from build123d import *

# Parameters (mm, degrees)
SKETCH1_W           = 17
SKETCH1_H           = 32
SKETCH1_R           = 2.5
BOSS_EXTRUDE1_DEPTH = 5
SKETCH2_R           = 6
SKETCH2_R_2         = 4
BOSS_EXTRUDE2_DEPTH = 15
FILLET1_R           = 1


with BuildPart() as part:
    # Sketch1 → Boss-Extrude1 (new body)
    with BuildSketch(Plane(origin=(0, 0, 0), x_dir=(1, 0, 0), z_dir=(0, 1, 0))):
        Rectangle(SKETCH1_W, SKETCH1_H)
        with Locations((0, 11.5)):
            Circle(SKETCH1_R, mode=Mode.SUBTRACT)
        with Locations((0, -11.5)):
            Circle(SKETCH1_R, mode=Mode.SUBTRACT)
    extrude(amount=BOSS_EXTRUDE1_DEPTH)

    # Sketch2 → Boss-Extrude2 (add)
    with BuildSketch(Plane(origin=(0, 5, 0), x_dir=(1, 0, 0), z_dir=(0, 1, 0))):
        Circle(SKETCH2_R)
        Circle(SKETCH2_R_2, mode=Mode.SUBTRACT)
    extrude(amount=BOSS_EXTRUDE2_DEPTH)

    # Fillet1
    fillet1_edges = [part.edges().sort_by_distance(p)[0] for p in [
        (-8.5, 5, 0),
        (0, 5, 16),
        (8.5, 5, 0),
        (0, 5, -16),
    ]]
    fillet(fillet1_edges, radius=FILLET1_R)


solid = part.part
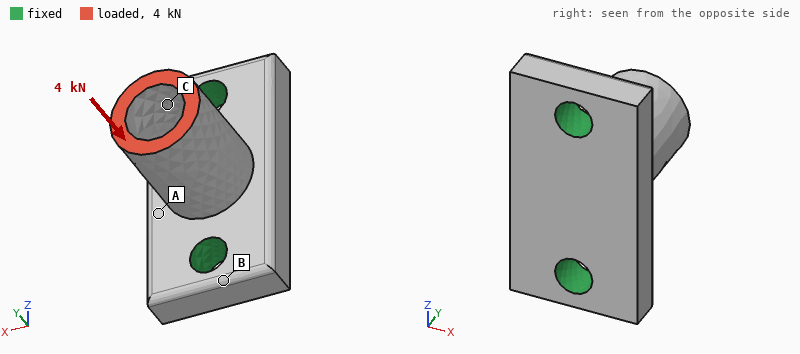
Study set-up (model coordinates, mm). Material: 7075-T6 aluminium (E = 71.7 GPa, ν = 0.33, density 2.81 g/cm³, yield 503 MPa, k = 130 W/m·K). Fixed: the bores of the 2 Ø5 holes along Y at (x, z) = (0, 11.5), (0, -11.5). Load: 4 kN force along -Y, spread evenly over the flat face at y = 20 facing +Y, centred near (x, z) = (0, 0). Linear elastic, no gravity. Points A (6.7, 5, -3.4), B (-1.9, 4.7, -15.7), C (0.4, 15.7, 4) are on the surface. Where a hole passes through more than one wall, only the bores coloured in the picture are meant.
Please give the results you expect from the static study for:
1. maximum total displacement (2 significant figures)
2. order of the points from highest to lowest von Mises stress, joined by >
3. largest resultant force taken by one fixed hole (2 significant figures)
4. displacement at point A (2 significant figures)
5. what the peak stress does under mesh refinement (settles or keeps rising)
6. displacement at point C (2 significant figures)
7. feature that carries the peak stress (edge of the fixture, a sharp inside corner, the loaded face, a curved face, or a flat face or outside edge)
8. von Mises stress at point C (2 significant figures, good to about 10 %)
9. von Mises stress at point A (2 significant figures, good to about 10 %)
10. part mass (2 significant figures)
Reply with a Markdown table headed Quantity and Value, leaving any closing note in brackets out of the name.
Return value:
| Quantity | Value |
|---|---|
| maximum total displacement | 28 µm |
| order of the points from highest to lowest von Mises stress, joined by > | C > A > B |
| largest resultant force taken by one fixed hole | 2.0 kN |
| displacement at point A | 15 µm |
| what the peak stress does under mesh refinement | keeps rising |
| displacement at point C | 24 µm |
| feature that carries the peak stress | edge of the fixture |
| von Mises stress at point C | 71 MPa |
| von Mises stress at point A | 43 MPa |
| part mass | 9.7 g |
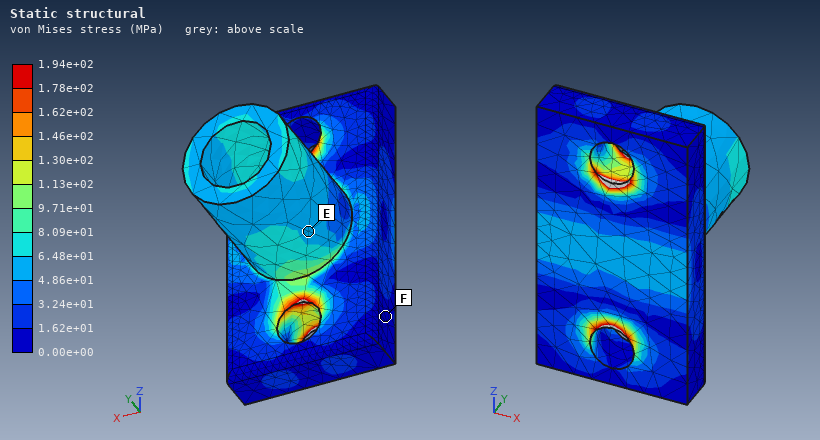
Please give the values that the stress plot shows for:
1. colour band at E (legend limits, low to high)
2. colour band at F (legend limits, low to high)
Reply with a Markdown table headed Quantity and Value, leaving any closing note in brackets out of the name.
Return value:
| Quantity | Value |
|---|---|
| colour band at E | 4.86e+01 to 6.48e+01 MPa |
| colour band at F | 0.00e+00 to 1.62e+01 MPa |
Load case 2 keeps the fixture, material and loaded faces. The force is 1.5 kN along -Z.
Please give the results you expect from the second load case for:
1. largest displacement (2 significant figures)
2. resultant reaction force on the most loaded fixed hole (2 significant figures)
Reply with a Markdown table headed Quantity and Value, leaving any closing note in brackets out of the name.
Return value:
| Quantity | Value |
|---|---|
| largest displacement | 87 µm |
| resultant reaction force on the most loaded fixed hole | 1.7 kN |
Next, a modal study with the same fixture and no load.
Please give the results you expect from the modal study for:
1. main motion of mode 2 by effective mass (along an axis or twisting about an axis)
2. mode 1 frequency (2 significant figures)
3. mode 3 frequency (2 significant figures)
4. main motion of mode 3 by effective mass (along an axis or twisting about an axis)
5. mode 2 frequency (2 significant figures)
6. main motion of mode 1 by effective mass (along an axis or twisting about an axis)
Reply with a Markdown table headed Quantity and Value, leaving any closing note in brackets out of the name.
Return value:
| Quantity | Value |
|---|---|
| main motion of mode 2 by effective mass | along Z |
| mode 1 frequency | 15 kHz |
| mode 3 frequency | 33 kHz |
| main motion of mode 3 by effective mass | along Y |
| mode 2 frequency | 23 kHz |
| main motion of mode 1 by effective mass | along X |
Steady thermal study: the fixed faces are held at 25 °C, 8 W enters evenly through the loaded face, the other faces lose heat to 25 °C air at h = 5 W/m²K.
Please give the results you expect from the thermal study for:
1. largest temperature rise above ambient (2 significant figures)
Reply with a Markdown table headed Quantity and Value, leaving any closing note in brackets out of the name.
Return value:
| Quantity | Value |
|---|---|
| largest temperature rise above ambient | 18 K |
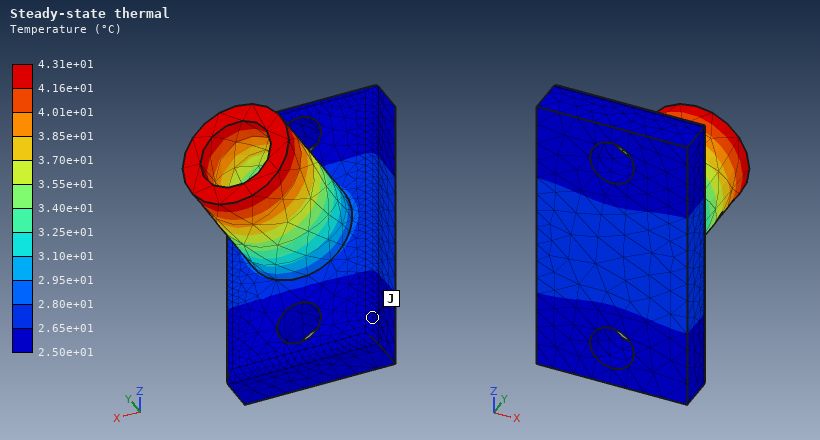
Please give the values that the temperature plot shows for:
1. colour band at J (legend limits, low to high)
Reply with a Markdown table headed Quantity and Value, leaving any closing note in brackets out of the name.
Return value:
| Quantity | Value |
|---|---|
| colour band at J | 2.50e+01 to 2.65e+01 °C |
